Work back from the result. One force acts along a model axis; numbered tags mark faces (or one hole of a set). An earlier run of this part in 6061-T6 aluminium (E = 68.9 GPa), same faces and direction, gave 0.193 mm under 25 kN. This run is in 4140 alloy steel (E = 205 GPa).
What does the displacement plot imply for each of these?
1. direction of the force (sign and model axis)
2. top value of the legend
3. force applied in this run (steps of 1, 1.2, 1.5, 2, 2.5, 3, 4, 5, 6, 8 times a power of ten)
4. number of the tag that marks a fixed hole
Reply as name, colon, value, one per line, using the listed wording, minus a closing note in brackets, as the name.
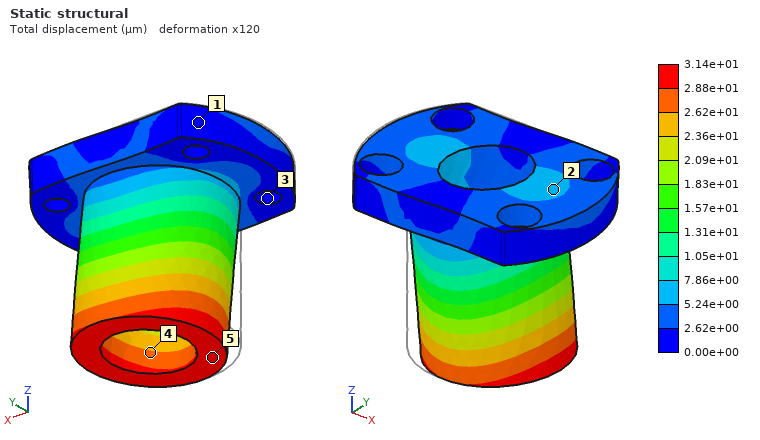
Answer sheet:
direction of the force: +X
top value of the legend: 3.14e+01 µm
force applied in this run: 12 kN
number of the tag that marks a fixed hole: 3
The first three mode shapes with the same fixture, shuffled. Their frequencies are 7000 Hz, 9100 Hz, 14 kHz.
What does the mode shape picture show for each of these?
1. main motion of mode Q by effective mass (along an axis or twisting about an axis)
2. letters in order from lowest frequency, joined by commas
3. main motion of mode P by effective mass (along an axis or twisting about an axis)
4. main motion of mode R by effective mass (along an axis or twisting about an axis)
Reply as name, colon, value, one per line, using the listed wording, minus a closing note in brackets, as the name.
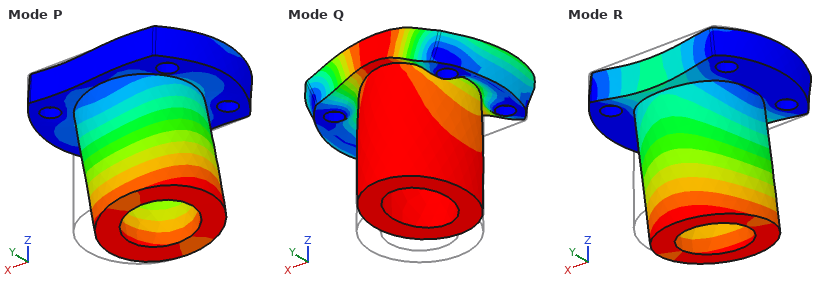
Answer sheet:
main motion of mode Q by effective mass: along Z
letters in order from lowest frequency, joined by commas: R, P, Q
main motion of mode P by effective mass: along X
main motion of mode R by effective mass: along Y
